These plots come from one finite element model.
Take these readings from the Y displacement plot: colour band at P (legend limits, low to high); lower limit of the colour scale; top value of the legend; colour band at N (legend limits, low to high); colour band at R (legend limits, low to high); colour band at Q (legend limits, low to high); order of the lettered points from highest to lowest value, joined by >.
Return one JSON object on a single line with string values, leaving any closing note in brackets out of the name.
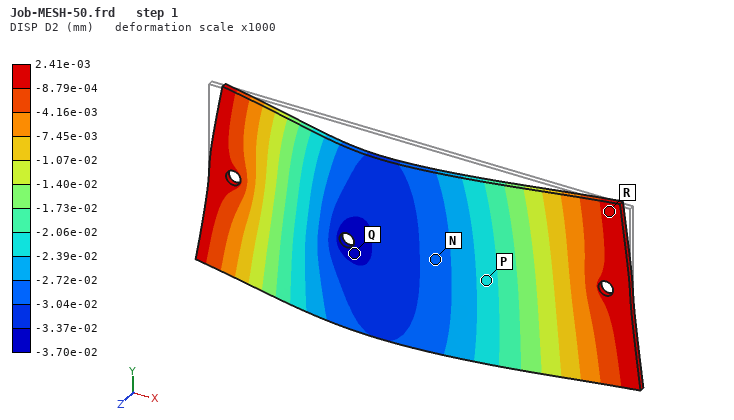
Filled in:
{"colour band at P": "-2.39e-02 to -2.06e-02 mm", "lower limit of the colour scale": "-3.70e-02 mm", "top value of the legend": "2.41e-03 mm", "colour band at N": "-3.04e-02 to -2.72e-02 mm", "colour band at R": "-8.79e-04 to 2.41e-03 mm", "colour band at Q": "-3.70e-02 to -3.37e-02 mm", "order of the lettered points from highest to lowest value, joined by >": "R > P > N > Q"}
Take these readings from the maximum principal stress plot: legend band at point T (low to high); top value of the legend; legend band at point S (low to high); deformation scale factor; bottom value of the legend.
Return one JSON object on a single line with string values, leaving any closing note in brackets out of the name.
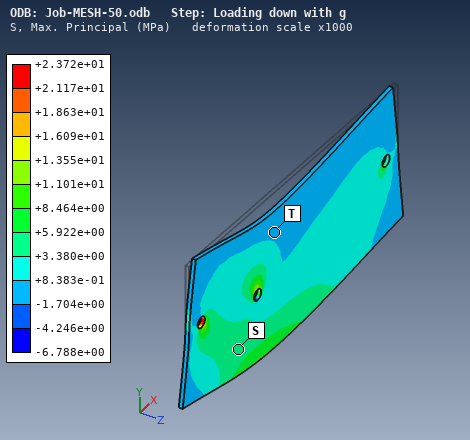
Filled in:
{"legend band at point T": "-1.704e+00 to +8.383e-01 MPa", "top value of the legend": "+2.372e+01 MPa", "legend band at point S": "+3.380e+00 to +5.922e+00 MPa", "deformation scale factor": "1000", "bottom value of the legend": "-6.788e+00 MPa"}
